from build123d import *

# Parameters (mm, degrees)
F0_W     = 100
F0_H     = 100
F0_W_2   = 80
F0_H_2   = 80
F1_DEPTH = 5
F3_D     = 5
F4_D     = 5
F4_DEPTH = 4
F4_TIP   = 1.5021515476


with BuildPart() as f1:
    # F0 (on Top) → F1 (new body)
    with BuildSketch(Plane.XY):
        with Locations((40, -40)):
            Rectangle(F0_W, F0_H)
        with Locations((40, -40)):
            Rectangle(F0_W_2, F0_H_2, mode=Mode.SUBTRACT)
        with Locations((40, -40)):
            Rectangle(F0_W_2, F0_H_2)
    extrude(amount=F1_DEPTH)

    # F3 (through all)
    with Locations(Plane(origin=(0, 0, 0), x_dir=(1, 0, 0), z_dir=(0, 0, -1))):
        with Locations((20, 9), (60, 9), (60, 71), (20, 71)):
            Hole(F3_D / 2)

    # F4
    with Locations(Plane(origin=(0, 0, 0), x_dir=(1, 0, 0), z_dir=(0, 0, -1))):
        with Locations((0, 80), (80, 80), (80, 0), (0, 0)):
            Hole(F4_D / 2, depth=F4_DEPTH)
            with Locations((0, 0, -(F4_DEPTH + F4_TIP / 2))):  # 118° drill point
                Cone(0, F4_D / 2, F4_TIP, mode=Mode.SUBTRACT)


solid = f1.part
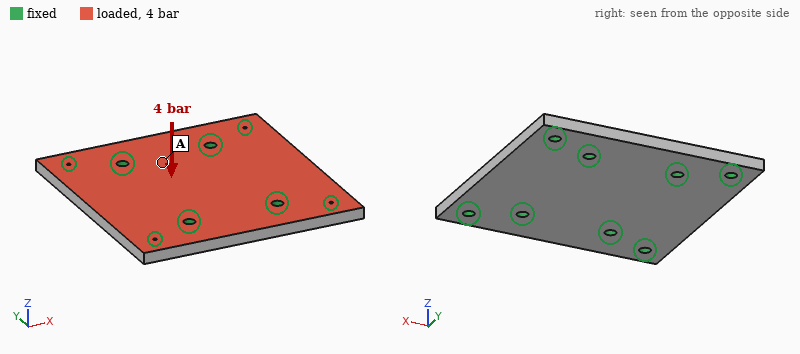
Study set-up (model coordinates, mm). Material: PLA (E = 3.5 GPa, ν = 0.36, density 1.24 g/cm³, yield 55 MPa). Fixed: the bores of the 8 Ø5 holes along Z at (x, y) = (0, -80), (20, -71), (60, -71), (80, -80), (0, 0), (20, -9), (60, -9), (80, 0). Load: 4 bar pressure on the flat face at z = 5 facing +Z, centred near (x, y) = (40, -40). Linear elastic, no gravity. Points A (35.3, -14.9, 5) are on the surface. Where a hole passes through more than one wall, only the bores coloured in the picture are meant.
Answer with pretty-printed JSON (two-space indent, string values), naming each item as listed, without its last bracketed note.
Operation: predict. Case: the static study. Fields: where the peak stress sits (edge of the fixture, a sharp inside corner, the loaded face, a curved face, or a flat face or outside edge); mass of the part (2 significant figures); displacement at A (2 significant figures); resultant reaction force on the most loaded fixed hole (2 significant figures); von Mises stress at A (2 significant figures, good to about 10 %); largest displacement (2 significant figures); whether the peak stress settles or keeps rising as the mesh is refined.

{
  "where the peak stress sits": "edge of the fixture",
  "mass of the part": "61 g",
  "displacement at A": "0.17 mm",
  "resultant reaction force on the most loaded fixed hole": "700 N",
  "von Mises stress at A": "10 MPa",
  "largest displacement": "0.95 mm",
  "whether the peak stress settles or keeps rising as the mesh is refined": "keeps rising"
}
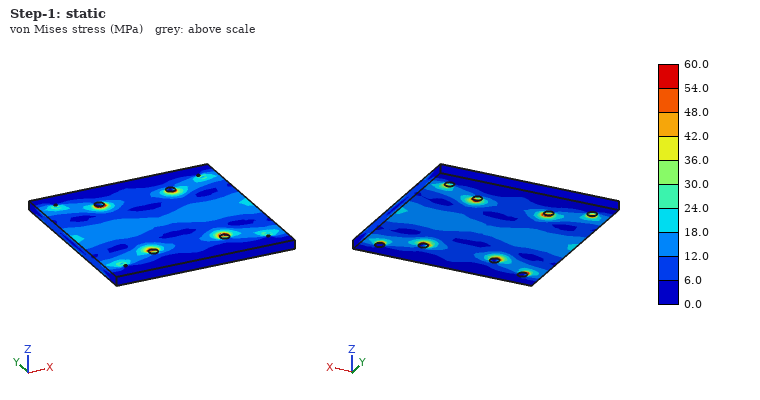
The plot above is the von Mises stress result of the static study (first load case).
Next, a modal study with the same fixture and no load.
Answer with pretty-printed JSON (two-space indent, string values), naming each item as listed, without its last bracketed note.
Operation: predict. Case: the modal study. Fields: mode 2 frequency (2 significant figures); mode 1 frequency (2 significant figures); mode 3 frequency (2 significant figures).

{
  "mode 2 frequency": "1700 Hz",
  "mode 1 frequency": "1700 Hz",
  "mode 3 frequency": "2400 Hz"
}
